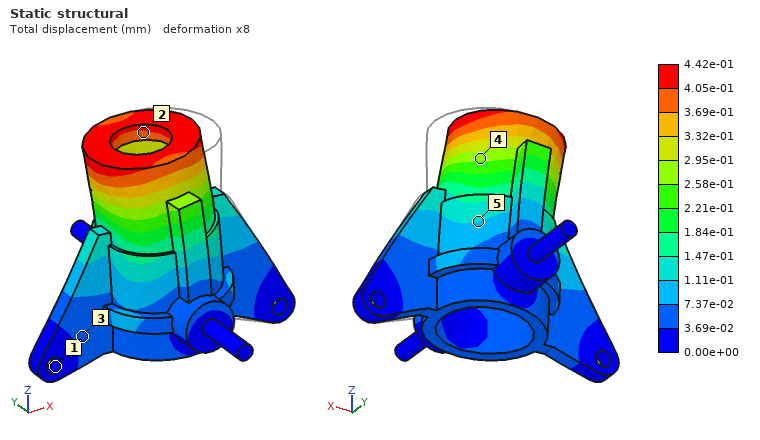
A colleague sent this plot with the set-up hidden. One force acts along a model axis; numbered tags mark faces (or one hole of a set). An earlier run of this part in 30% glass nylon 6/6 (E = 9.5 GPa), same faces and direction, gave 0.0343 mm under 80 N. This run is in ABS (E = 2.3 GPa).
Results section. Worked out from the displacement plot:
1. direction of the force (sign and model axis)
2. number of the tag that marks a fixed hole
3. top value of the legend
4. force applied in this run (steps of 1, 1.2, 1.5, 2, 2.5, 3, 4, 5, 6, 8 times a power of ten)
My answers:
-X
1
4.42e-01 mm
250 N
